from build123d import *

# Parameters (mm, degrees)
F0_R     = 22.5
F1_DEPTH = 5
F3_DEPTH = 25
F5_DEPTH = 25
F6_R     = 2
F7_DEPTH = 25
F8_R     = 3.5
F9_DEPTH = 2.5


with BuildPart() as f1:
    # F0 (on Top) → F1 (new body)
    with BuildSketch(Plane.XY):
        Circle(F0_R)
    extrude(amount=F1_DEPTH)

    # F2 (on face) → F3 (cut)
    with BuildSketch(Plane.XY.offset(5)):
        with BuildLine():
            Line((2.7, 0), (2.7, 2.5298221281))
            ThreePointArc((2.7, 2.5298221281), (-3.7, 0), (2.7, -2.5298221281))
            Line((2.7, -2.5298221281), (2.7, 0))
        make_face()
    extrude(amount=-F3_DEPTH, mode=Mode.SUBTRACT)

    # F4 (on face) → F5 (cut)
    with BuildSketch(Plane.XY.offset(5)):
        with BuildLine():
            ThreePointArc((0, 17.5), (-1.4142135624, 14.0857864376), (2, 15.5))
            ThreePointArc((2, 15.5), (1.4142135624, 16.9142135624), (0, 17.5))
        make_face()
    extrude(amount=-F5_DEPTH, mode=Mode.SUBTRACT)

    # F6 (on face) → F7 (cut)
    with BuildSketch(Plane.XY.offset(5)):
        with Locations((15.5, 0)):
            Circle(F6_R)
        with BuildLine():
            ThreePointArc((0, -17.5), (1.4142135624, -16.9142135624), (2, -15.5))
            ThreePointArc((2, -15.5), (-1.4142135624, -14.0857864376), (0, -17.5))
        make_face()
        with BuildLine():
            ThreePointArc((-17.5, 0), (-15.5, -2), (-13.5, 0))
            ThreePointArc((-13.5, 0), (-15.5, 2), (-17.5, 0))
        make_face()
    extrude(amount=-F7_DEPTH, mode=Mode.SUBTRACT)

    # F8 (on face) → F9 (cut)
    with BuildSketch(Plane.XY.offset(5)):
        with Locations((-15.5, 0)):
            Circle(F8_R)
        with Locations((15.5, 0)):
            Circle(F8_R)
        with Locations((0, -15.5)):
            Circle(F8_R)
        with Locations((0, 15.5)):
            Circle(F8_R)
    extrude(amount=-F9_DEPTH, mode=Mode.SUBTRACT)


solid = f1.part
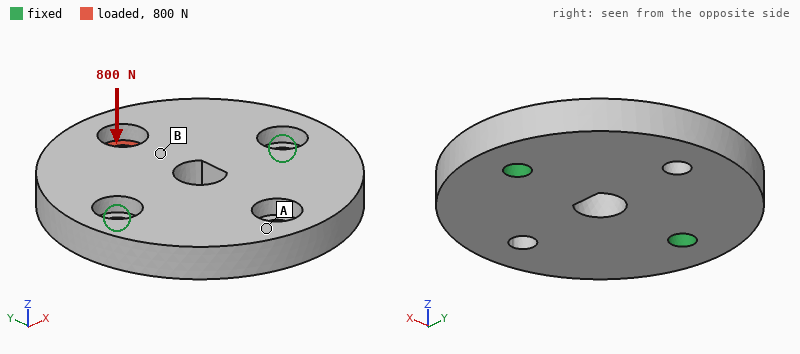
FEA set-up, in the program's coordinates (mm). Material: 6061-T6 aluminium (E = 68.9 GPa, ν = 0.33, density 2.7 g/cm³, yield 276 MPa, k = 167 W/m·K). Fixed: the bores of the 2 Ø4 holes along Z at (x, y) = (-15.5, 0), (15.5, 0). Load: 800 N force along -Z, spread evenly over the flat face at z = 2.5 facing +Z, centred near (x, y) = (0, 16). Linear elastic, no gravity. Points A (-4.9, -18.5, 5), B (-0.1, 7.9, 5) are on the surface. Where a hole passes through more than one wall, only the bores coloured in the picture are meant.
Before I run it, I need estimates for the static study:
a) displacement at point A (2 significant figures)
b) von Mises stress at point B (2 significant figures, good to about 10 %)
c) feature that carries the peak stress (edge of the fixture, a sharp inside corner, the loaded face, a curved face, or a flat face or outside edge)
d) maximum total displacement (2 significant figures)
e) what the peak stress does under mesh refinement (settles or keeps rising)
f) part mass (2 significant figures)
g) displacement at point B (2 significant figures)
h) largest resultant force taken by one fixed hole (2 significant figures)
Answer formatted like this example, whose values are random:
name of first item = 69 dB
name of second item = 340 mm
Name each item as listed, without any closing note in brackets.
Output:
displacement at point A = 0.063 mm
von Mises stress at point B = 57 MPa
feature that carries the peak stress = edge of the fixture
maximum total displacement = 0.18 mm
what the peak stress does under mesh refinement = keeps rising
part mass = 20 g
displacement at point B = 0.067 mm
largest resultant force taken by one fixed hole = 540 N
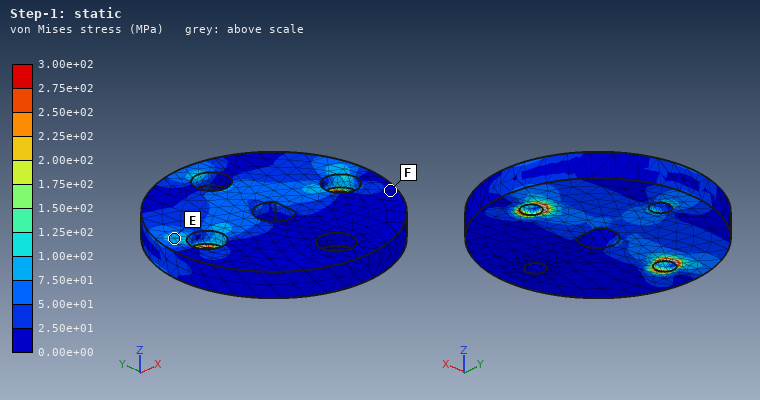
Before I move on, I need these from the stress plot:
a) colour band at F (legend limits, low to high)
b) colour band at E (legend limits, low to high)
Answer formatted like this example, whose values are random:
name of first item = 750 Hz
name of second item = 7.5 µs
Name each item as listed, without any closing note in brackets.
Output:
colour band at F = 0.00e+00 to 2.50e+01 MPa
colour band at E = 7.50e+01 to 1.00e+02 MPa
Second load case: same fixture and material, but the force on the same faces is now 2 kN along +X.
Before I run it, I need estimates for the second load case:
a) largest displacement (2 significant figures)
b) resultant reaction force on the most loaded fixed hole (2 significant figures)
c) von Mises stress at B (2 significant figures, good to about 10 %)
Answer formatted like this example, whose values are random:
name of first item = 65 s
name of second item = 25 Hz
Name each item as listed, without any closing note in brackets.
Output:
largest displacement = 17 µm
resultant reaction force on the most loaded fixed hole = 1.4 kN
von Mises stress at B = 33 MPa
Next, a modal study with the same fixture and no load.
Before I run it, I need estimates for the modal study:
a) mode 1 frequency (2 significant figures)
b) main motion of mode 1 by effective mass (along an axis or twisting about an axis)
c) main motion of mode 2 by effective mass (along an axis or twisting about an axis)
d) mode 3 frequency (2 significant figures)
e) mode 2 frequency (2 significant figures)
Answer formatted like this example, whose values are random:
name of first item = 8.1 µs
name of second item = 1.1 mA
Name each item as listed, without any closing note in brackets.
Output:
mode 1 frequency = 5000 Hz
main motion of mode 1 by effective mass = twisting about X
main motion of mode 2 by effective mass = along Z
mode 3 frequency = 14 kHz
mode 2 frequency = 8400 Hz
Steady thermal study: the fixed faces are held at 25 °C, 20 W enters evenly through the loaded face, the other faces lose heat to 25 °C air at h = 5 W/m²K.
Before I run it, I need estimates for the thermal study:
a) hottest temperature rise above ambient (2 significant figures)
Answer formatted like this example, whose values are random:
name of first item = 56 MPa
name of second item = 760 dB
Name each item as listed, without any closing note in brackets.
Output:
hottest temperature rise above ambient = 25 K
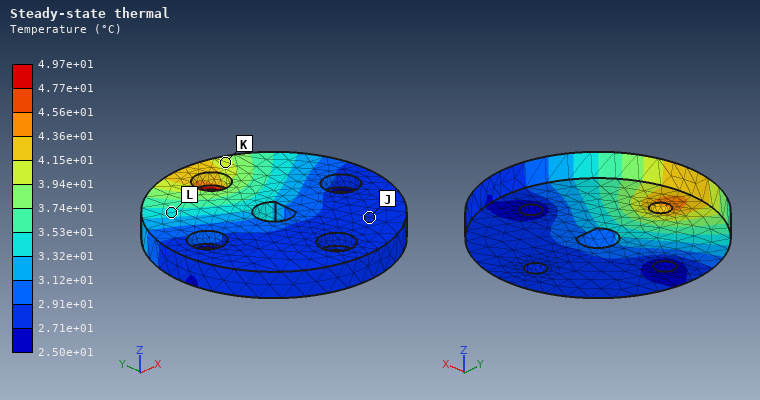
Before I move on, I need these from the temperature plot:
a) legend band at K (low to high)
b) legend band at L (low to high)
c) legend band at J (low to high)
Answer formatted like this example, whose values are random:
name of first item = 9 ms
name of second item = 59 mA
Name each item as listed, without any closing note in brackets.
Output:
legend band at K = 3.94e+01 to 4.15e+01 °C
legend band at L = 3.32e+01 to 3.53e+01 °C
legend band at J = 2.71e+01 to 2.91e+01 °C
